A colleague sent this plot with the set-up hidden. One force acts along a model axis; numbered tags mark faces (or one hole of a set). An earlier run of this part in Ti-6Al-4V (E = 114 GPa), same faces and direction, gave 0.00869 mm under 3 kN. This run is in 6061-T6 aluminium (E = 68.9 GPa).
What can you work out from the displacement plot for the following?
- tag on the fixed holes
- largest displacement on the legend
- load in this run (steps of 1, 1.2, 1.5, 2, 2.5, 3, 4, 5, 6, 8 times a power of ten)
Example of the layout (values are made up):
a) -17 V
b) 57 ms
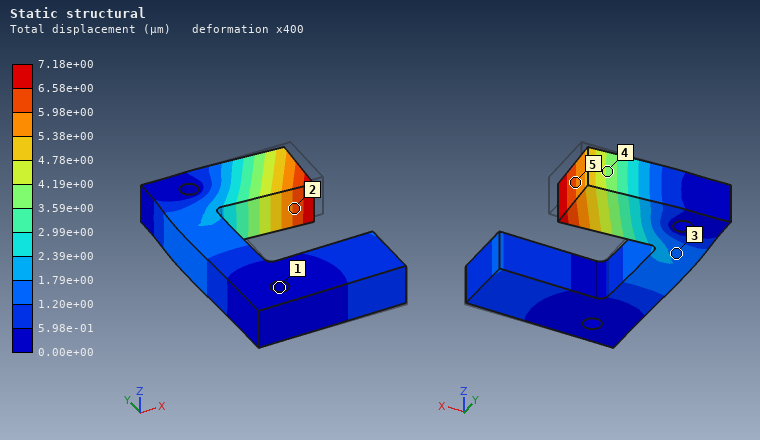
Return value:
a) 1
b) 7.18e+00 µm
c) 1.5 kN
